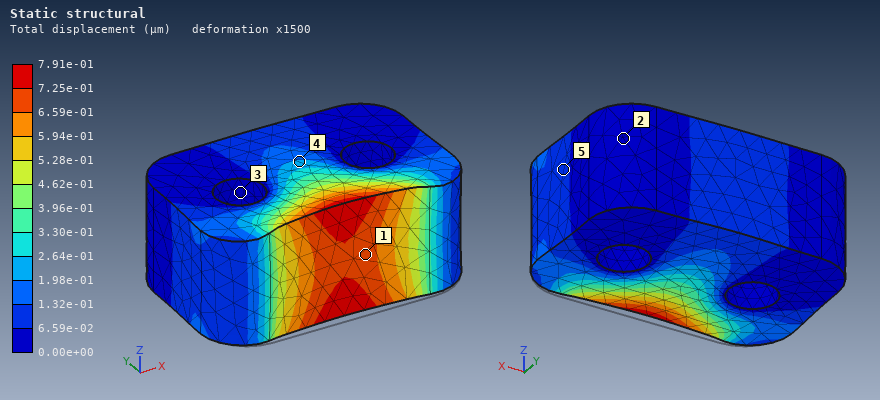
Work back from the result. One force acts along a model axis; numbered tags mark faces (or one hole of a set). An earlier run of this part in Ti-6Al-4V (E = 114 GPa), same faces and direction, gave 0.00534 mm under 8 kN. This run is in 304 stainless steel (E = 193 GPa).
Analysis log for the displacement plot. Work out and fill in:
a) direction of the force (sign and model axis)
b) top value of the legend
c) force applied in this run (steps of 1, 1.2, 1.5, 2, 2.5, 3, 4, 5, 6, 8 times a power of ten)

+Y
7.91e-01 µm
2 kN
